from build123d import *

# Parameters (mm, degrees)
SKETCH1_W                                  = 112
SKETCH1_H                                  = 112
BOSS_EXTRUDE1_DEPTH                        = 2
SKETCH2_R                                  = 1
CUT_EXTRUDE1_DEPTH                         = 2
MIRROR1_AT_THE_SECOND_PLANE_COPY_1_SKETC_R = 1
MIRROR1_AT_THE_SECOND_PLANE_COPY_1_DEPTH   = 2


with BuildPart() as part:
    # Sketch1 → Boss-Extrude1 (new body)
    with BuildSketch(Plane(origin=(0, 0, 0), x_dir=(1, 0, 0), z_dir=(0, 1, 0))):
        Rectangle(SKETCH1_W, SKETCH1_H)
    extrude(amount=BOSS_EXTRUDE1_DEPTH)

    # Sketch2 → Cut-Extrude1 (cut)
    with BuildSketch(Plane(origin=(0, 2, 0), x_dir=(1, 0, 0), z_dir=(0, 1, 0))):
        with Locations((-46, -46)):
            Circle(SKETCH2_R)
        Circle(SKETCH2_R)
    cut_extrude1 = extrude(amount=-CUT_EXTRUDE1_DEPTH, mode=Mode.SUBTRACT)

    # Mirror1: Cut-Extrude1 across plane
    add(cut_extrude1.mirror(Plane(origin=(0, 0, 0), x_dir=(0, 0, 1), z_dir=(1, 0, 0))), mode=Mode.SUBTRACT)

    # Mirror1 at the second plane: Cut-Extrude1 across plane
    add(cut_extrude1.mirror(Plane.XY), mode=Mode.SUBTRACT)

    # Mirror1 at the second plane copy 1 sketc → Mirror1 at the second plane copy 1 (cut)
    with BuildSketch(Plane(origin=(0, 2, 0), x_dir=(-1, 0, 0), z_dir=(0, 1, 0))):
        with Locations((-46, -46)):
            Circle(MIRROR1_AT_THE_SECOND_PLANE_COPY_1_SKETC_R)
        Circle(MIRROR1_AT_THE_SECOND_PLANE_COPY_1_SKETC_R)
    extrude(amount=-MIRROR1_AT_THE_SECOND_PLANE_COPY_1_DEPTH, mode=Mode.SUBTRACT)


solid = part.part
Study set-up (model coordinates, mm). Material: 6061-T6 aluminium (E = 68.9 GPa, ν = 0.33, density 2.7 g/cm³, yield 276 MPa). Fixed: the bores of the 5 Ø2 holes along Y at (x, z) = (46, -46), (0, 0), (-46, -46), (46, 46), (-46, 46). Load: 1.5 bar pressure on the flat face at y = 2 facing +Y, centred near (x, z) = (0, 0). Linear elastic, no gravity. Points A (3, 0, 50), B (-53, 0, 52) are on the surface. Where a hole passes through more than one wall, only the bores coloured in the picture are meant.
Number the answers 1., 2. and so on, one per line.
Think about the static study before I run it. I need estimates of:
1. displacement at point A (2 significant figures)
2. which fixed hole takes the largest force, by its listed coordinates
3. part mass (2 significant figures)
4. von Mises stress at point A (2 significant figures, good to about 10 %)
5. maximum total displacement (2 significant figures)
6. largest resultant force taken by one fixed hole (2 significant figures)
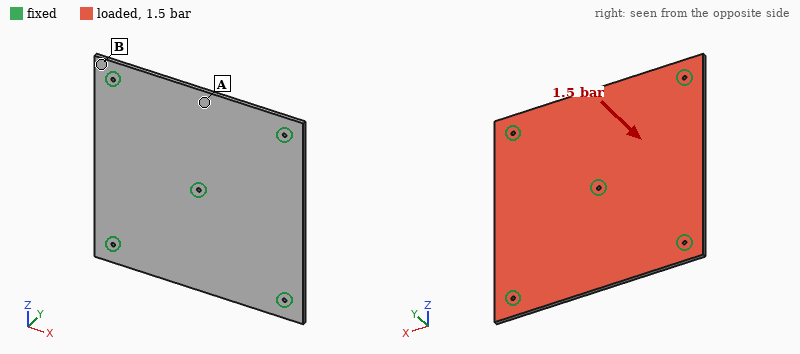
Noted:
1. 0.44 mm
2. (0, 0)
3. 68 g
4. 48 MPa
5. 0.49 mm
6. 690 N
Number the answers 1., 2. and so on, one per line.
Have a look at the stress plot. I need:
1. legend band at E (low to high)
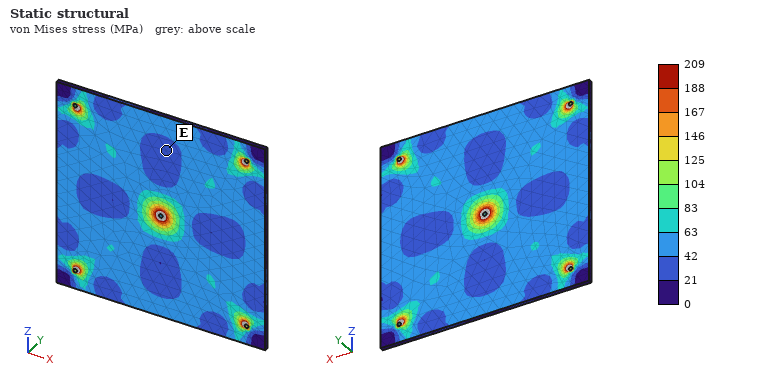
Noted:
1. 21 to 42 MPa
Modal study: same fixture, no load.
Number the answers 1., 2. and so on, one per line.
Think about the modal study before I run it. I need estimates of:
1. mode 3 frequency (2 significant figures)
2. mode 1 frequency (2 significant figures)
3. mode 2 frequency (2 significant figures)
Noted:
1. 1400 Hz
2. 1300 Hz
3. 1400 Hz
